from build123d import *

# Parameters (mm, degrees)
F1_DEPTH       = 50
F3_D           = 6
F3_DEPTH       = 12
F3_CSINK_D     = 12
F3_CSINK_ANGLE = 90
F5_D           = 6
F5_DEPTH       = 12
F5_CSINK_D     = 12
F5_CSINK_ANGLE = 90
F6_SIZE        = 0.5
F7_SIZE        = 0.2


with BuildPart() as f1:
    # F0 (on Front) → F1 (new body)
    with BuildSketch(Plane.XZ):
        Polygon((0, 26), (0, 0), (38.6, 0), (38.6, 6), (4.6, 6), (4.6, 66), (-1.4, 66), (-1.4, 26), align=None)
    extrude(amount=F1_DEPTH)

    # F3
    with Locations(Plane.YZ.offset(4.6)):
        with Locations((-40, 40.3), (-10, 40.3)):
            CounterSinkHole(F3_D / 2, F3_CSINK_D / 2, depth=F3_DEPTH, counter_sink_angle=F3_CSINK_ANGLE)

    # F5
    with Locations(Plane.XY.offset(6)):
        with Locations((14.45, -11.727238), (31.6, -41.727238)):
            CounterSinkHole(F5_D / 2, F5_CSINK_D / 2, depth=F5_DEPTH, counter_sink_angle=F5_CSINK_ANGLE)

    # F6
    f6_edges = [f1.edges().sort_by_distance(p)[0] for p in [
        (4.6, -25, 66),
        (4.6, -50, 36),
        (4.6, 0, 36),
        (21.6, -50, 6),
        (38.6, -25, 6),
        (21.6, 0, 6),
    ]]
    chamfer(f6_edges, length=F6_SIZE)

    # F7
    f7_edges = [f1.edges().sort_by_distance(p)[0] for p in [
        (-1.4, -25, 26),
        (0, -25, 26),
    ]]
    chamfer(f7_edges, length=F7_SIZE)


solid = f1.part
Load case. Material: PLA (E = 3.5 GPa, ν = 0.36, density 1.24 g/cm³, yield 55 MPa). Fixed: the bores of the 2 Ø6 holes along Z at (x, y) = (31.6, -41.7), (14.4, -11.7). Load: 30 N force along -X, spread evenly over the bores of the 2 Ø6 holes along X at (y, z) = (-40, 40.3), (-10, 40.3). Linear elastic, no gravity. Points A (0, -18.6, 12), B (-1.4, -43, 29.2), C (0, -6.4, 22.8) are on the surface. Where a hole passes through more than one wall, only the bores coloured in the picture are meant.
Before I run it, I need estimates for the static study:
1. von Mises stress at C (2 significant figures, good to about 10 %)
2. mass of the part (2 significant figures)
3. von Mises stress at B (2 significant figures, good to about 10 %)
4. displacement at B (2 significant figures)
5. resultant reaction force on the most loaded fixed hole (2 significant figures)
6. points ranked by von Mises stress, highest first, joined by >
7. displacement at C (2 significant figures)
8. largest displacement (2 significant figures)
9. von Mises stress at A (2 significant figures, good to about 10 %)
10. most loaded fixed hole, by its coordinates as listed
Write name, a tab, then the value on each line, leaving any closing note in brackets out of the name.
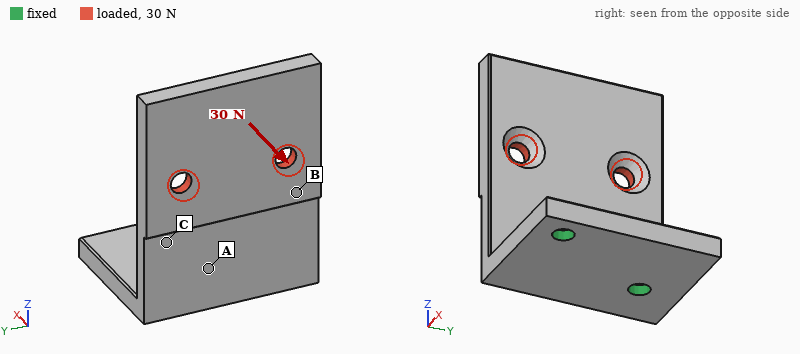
von Mises stress at C	2.9 MPa
mass of the part	33 g
von Mises stress at B	1.1 MPa
displacement at B	0.40 mm
resultant reaction force on the most loaded fixed hole	23 N
points ranked by von Mises stress, highest first, joined by >	A > C > B
displacement at C	0.25 mm
largest displacement	1.1 mm
von Mises stress at A	4.3 MPa
most loaded fixed hole, by its coordinates as listed	(31.6, -41.7)
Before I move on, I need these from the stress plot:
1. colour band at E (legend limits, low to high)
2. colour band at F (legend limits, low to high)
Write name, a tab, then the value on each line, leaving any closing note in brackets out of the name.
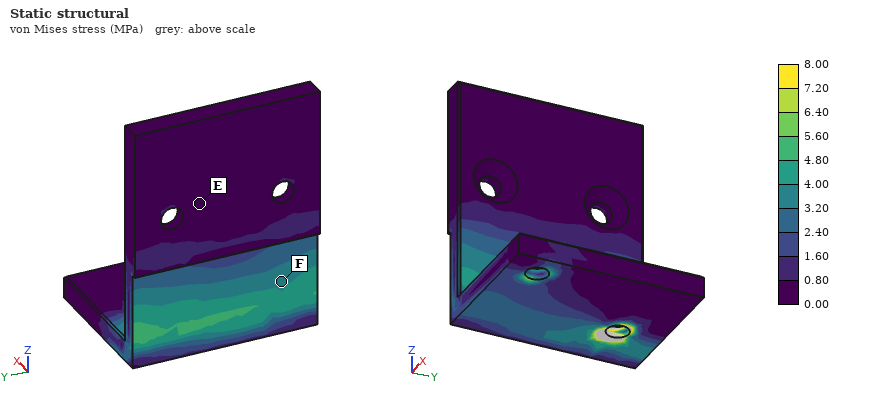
colour band at E	0.00 to 0.80 MPa
colour band at F	3.20 to 4.00 MPa
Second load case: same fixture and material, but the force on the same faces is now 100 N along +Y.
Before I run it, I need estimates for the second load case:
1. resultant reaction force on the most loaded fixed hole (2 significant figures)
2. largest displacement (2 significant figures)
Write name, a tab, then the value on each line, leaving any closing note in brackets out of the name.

resultant reaction force on the most loaded fixed hole	130 N
largest displacement	0.94 mm
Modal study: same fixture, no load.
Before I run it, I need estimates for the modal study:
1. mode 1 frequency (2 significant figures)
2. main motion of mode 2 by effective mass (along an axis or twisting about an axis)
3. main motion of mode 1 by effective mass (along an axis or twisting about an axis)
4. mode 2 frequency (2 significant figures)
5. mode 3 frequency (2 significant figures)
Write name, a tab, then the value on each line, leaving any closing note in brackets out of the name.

mode 1 frequency	230 Hz
main motion of mode 2 by effective mass	along Y
main motion of mode 1 by effective mass	along X
mode 2 frequency	490 Hz
mode 3 frequency	910 Hz
